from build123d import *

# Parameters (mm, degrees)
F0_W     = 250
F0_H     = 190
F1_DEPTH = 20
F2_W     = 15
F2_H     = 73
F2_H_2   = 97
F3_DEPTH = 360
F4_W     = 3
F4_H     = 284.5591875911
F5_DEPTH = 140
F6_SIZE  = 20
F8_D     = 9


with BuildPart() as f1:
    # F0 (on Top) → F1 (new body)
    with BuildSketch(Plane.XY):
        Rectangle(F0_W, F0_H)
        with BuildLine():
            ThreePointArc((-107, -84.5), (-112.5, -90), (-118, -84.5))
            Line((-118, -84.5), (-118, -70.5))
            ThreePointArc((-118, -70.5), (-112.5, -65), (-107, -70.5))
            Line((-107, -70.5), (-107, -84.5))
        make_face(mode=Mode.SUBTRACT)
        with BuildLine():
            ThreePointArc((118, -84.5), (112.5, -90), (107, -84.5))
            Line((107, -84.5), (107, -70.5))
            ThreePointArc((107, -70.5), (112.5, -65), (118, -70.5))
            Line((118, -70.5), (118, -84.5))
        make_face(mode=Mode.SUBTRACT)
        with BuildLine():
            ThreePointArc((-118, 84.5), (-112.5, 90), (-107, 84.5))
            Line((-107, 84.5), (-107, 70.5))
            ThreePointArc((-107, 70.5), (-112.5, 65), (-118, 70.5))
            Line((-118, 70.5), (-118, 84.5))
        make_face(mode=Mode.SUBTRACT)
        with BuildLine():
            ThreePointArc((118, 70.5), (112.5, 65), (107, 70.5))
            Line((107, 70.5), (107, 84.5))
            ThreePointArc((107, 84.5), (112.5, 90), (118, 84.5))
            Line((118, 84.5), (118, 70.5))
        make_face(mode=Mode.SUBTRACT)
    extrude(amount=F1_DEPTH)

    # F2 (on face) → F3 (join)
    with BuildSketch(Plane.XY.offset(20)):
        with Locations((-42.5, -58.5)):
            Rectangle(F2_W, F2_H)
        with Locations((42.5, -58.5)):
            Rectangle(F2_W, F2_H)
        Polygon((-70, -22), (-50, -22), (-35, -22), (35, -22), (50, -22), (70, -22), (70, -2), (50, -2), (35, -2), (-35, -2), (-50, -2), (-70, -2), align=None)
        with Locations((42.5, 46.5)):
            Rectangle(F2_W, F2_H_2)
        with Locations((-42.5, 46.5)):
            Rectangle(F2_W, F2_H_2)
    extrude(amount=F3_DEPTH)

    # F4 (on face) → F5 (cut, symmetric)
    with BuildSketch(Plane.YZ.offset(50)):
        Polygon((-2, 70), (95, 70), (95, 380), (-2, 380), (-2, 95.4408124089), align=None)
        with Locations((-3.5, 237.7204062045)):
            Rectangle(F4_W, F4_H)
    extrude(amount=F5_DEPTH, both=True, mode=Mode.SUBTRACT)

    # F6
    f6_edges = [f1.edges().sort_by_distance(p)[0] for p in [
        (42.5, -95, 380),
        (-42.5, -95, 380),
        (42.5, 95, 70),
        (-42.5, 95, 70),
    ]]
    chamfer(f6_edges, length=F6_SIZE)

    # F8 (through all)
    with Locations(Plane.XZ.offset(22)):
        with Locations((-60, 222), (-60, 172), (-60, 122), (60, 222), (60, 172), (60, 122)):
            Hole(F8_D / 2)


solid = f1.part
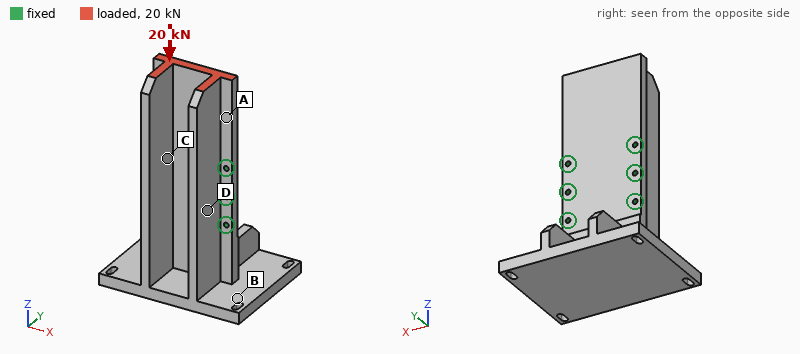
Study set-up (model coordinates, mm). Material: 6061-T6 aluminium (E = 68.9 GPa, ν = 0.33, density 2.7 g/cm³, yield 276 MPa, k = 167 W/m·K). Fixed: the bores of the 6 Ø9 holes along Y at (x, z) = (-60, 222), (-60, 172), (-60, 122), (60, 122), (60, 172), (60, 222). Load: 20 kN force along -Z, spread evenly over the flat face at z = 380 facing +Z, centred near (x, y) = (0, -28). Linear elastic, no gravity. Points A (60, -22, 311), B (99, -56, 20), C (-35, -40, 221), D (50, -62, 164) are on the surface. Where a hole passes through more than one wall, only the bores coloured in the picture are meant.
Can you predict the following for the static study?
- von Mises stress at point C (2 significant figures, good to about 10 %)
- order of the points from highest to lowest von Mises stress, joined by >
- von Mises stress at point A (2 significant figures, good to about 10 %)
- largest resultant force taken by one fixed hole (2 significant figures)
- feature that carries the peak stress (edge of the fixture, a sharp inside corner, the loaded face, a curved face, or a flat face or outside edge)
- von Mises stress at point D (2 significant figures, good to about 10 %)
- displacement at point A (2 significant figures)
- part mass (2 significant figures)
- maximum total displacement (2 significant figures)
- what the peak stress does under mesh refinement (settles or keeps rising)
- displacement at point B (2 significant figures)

3.7 MPa
A > C > D > B
5.0 MPa
5.9 kN
edge of the fixture
2.2 MPa
13 µm
7.4 kg
19 µm
keeps rising
12 µm
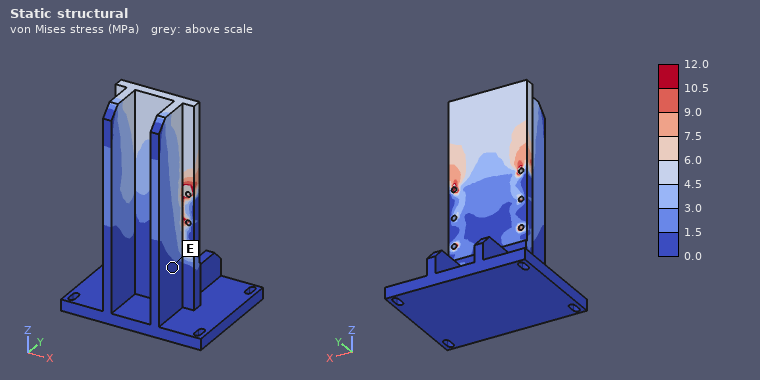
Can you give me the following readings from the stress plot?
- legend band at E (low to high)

0.0 to 1.5 MPa
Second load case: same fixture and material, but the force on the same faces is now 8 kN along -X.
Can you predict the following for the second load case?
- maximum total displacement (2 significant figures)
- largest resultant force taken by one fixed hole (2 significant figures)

0.15 mm
10 kN
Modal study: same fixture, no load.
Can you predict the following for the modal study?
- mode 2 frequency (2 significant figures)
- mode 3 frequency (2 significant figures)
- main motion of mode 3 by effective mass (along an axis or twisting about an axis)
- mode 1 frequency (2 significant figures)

730 Hz
1300 Hz
along X
720 Hz
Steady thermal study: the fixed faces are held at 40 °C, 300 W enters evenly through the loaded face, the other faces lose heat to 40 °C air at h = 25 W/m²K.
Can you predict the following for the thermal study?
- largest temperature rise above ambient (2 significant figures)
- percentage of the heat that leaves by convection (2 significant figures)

64 K
31 %
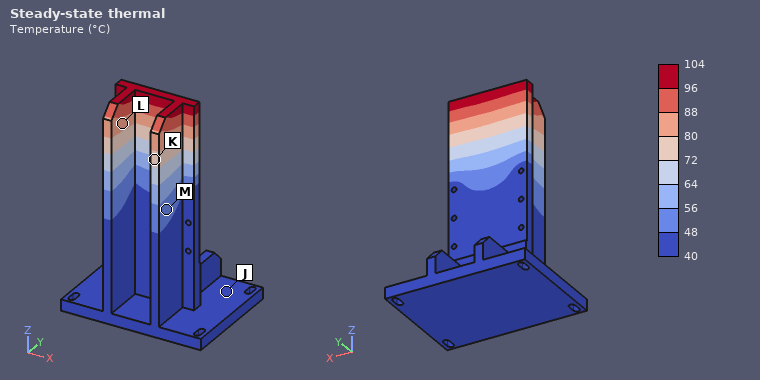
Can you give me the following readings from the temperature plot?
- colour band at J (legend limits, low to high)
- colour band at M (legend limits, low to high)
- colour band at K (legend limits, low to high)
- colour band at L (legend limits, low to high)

40 to 48 °C
48 to 56 °C
72 to 80 °C
80 to 88 °C
